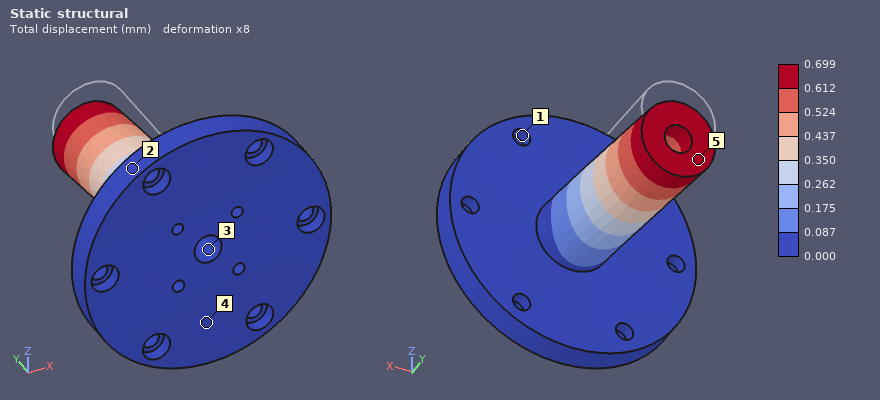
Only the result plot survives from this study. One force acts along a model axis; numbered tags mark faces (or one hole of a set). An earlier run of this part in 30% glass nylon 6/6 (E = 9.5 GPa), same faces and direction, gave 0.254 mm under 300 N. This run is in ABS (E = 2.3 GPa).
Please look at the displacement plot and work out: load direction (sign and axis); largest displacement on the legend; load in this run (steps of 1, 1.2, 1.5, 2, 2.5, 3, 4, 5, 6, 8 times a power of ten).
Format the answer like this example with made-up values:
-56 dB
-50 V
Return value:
-Z
0.699 mm
200 N
